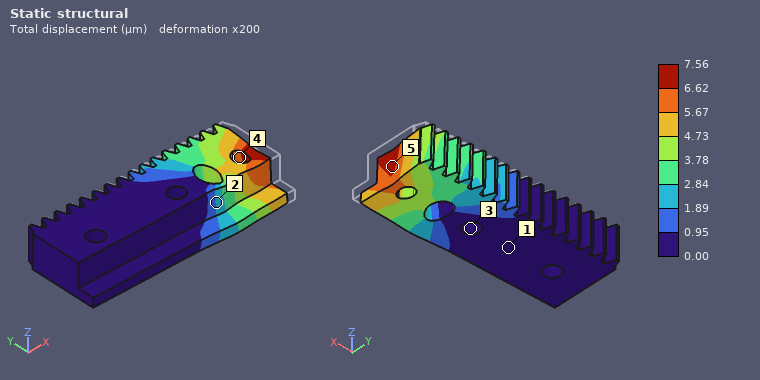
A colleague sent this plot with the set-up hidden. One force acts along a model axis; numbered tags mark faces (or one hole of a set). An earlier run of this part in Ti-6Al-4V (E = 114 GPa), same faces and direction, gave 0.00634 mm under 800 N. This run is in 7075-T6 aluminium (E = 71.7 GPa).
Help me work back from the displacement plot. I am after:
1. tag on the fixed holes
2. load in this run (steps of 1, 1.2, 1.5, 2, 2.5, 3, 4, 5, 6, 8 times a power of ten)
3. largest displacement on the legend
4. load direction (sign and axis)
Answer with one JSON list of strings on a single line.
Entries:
["3", "600 N", "7.56 µm", "-X"]
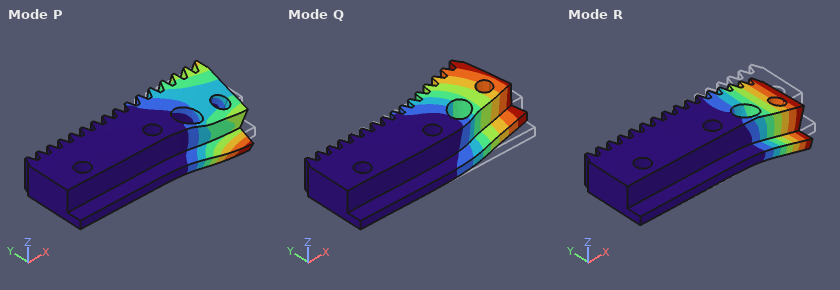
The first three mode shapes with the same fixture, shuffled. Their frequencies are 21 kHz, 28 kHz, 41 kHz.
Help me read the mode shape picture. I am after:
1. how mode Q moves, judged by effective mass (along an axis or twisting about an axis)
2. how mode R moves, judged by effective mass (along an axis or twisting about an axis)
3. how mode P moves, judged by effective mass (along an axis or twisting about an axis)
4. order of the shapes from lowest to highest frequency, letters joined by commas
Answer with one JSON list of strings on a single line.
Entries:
["along Y", "along Z", "twisting about X", "R, Q, P"]
